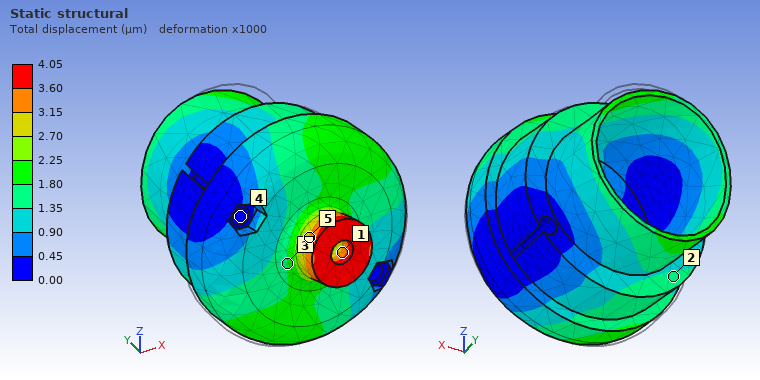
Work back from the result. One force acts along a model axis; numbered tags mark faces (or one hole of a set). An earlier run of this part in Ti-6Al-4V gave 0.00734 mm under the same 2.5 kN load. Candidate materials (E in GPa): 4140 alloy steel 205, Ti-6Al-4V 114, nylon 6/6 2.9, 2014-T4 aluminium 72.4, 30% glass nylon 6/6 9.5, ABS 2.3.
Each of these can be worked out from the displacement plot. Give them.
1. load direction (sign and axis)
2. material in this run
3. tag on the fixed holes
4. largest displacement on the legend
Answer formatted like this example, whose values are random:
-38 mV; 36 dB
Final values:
+Z; 4140 alloy steel; 4; 4.05 µm
